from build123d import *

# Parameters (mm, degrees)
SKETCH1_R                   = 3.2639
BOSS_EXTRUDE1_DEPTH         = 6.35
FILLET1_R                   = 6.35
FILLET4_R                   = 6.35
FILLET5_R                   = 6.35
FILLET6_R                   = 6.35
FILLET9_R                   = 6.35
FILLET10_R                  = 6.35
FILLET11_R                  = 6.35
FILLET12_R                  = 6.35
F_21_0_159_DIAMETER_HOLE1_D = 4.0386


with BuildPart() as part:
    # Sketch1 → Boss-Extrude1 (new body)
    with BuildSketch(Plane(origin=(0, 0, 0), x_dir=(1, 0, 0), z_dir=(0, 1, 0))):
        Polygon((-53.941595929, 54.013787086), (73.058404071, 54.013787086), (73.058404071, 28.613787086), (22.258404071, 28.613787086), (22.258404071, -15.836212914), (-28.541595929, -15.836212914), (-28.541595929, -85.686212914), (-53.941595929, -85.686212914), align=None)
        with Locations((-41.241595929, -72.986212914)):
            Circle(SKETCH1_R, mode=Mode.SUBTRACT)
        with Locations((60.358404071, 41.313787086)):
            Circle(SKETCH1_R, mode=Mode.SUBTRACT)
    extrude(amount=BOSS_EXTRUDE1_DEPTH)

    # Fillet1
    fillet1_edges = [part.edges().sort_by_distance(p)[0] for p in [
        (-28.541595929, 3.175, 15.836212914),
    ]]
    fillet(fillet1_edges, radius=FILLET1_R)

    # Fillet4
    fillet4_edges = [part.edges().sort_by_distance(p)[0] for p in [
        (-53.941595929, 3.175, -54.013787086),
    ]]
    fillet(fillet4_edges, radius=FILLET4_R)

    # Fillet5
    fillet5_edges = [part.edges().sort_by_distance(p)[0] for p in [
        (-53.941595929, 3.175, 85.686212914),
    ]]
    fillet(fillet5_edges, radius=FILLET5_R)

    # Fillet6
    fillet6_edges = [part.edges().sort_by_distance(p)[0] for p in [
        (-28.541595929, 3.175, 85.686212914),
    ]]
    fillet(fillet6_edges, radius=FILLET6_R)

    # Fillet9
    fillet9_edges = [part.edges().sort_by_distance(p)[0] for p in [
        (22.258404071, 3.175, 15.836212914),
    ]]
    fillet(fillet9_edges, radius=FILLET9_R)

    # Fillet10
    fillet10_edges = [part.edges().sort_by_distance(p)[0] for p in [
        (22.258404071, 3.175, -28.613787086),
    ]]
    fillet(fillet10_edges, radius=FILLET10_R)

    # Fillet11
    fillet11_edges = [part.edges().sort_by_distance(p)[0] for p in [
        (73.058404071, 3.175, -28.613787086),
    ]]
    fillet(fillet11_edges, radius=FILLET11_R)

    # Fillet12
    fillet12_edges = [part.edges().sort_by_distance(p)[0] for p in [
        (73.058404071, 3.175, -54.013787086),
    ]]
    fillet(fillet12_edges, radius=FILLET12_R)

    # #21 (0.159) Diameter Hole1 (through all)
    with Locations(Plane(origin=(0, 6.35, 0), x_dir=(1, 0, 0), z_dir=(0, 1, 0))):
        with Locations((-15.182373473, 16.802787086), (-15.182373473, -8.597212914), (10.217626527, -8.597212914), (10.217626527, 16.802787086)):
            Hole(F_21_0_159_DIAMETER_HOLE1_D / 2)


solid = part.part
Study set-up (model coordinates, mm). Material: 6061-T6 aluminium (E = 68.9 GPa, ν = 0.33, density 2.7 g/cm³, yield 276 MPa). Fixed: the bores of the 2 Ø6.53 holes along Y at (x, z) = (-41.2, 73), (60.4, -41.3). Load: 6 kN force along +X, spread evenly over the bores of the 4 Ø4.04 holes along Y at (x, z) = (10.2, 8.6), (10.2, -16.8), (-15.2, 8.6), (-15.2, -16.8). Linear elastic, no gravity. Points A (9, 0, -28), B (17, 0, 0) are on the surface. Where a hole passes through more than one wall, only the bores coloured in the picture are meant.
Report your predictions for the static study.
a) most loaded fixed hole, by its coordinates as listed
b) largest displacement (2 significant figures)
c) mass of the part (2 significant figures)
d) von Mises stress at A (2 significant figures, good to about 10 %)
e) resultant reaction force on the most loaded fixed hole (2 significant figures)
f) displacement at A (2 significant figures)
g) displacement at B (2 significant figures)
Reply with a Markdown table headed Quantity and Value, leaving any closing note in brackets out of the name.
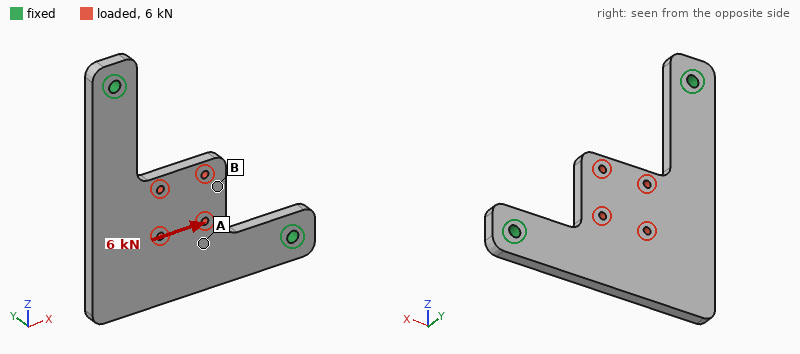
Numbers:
| Quantity | Value |
|---|---|
| most loaded fixed hole, by its coordinates as listed | (60.4, -41.3) |
| largest displacement | 85 µm |
| mass of the part | 140 g |
| von Mises stress at A | 32 MPa |
| resultant reaction force on the most loaded fixed hole | 5.3 kN |
| displacement at A | 36 µm |
| displacement at B | 70 µm |
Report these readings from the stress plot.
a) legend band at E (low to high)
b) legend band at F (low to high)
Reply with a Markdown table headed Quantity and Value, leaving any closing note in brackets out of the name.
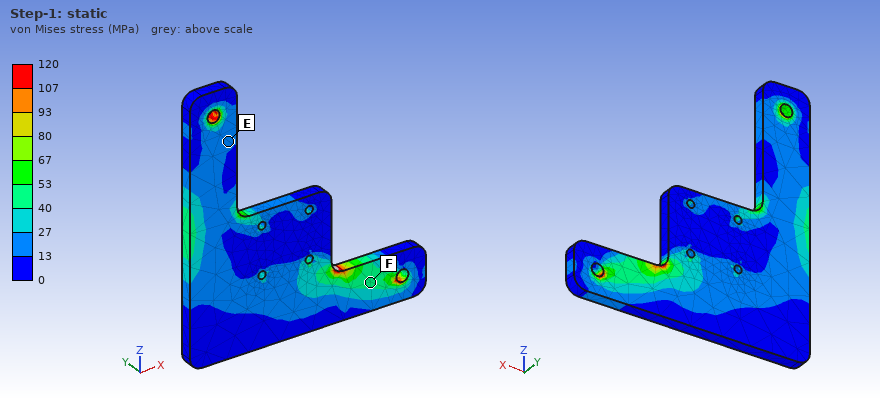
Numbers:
| Quantity | Value |
|---|---|
| legend band at E | 13 to 27 MPa |
| legend band at F | 40 to 53 MPa |
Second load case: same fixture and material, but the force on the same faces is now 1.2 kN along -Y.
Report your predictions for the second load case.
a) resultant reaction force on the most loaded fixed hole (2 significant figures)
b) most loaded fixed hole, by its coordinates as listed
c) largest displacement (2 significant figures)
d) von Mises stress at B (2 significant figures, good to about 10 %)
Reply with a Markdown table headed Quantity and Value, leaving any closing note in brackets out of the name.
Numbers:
| Quantity | Value |
|---|---|
| resultant reaction force on the most loaded fixed hole | 670 N |
| most loaded fixed hole, by its coordinates as listed | (60.4, -41.3) |
| largest displacement | 0.76 mm |
| von Mises stress at B | 36 MPa |
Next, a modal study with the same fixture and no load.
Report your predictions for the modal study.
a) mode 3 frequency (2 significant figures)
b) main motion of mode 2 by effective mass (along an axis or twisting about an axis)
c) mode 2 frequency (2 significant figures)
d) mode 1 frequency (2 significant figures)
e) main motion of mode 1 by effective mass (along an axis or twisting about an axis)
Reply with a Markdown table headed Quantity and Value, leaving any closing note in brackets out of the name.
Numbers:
| Quantity | Value |
|---|---|
| mode 3 frequency | 2200 Hz |
| main motion of mode 2 by effective mass | along Y |
| mode 2 frequency | 1500 Hz |
| mode 1 frequency | 540 Hz |
| main motion of mode 1 by effective mass | along Y |
